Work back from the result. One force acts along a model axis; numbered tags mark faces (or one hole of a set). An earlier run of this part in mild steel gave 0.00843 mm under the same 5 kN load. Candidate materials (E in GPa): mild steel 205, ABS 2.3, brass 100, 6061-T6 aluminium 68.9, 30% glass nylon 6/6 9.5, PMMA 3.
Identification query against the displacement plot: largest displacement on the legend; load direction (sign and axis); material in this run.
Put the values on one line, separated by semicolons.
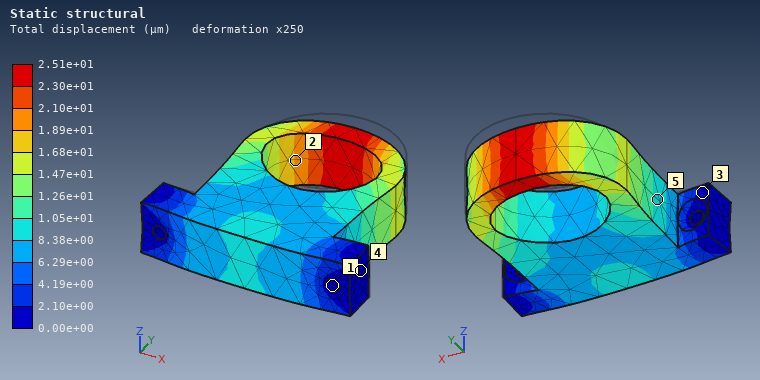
2.51e+01 µm; -Y; 6061-T6 aluminium
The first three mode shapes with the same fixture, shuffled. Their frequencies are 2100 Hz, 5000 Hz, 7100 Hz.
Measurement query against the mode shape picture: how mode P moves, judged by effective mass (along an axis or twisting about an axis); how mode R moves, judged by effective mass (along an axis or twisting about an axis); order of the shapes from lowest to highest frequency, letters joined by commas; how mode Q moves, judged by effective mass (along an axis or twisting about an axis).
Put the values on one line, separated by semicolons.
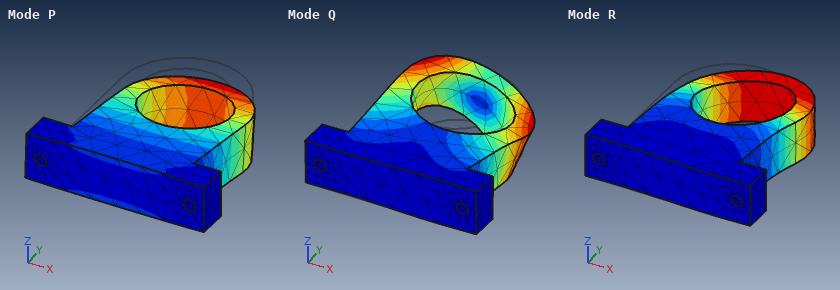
along Z; along X; P, R, Q; twisting about Y
